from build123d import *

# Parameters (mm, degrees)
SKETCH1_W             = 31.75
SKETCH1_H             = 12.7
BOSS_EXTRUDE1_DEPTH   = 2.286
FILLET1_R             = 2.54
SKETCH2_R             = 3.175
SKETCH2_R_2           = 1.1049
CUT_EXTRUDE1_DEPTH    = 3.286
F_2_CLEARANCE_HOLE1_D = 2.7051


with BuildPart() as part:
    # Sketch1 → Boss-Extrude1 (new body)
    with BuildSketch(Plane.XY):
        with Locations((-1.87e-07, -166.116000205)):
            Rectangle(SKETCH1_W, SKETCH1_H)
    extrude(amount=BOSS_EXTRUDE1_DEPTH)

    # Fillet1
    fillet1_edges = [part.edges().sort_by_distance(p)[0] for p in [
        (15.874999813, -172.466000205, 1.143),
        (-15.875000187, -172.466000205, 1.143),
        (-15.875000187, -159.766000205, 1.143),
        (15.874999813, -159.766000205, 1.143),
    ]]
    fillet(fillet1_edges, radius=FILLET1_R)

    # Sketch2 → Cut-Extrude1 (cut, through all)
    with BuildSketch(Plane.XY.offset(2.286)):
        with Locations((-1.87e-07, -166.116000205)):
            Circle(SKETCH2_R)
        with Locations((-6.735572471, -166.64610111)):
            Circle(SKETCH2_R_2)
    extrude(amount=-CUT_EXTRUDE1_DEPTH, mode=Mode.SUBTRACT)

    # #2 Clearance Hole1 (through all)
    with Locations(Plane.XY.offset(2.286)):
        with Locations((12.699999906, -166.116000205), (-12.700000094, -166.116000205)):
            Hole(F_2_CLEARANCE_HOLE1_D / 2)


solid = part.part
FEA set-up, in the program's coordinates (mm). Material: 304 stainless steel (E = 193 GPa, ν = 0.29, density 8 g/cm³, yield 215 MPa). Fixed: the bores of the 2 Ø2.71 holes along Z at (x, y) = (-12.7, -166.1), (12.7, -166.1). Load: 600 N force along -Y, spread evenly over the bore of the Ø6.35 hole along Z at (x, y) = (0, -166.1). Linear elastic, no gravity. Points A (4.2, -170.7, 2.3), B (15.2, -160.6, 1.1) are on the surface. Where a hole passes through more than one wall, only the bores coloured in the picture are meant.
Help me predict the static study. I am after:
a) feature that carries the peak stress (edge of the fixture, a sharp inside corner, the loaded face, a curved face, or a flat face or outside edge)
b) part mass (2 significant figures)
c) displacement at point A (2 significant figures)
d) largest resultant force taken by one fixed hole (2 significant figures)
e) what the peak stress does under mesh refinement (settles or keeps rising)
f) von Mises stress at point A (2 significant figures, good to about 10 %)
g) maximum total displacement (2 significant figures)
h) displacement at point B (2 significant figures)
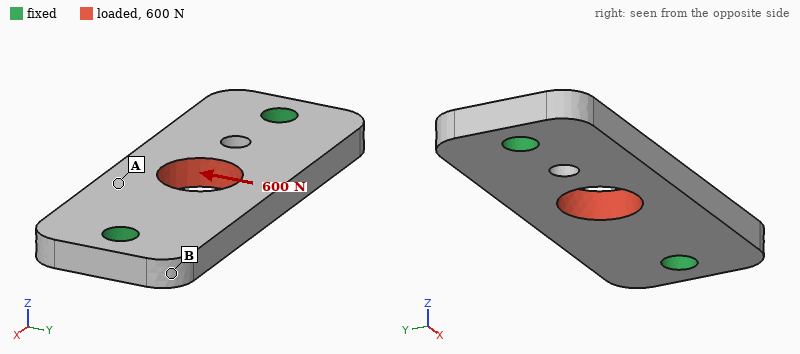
edge of the fixture
6.4 g
2.9 µm
300 N
keeps rising
24 MPa
3.7 µm
1.1 µm
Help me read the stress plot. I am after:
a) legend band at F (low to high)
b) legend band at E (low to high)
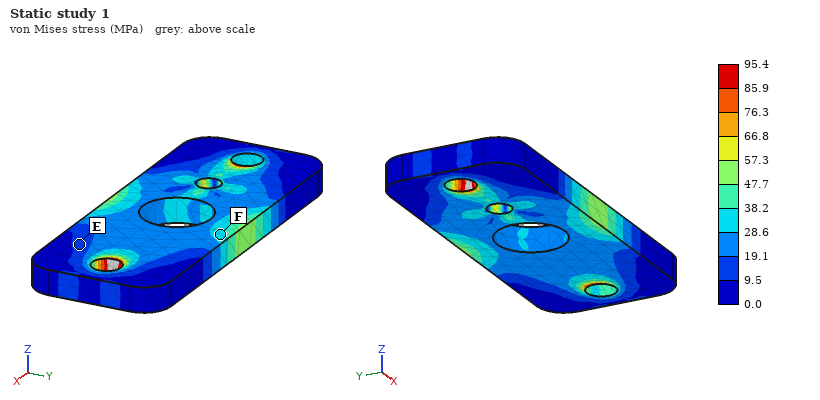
28.6 to 38.2 MPa
9.5 to 19.1 MPa
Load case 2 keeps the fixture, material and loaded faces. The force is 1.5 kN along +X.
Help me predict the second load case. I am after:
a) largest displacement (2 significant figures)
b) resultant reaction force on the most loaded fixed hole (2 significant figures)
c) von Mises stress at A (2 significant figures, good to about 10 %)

2.4 µm
770 N
23 MPa
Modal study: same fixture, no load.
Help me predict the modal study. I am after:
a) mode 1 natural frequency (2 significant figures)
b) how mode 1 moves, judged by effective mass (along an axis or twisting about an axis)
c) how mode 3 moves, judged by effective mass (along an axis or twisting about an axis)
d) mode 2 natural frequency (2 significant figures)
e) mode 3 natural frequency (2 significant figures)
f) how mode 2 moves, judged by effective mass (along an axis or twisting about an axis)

17 kHz
along Z
twisting about Y
21 kHz
39 kHz
twisting about X
